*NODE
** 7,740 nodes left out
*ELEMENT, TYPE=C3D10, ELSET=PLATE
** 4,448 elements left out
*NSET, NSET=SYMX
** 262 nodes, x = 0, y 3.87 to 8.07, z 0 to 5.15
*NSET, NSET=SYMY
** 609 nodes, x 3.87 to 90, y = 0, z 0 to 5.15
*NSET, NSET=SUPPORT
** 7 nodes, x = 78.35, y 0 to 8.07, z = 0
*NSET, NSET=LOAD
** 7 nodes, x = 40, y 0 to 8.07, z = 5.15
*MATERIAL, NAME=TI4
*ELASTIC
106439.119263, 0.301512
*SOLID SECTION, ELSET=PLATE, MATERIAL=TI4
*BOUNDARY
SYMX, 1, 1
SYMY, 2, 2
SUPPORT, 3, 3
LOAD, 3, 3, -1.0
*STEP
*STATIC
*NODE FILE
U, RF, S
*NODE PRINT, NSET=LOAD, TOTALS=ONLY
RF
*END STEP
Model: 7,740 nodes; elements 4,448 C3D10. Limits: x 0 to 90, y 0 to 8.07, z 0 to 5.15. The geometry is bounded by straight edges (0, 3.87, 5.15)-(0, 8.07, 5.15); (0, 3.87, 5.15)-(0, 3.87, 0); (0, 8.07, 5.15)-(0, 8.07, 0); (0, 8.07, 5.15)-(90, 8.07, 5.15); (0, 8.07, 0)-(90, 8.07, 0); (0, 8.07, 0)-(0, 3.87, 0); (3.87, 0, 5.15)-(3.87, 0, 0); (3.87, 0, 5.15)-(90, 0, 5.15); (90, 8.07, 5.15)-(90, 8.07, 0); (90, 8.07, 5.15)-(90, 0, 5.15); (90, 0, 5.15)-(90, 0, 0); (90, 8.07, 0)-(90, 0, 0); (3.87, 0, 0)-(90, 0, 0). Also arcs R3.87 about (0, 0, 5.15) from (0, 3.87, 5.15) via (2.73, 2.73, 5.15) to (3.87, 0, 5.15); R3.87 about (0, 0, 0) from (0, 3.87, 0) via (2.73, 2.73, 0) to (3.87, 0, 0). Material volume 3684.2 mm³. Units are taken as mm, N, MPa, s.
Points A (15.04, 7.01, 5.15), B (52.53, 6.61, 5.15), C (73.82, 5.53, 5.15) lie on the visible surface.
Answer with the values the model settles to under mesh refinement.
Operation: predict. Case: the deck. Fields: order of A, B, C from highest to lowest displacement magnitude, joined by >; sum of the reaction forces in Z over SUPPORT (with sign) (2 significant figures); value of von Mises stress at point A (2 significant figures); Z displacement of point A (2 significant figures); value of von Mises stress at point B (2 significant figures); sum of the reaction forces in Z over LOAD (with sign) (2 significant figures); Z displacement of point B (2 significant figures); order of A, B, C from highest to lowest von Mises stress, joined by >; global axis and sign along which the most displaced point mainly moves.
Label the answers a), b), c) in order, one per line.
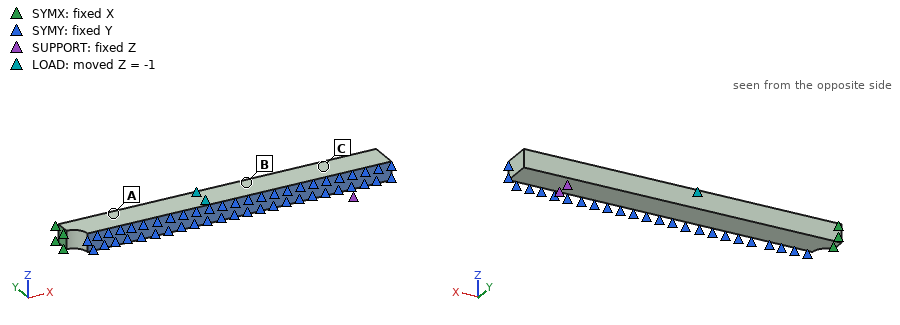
a) A > B > C
b) 120 N
c) 130 MPa
d) -1.4 mm
e) 85 MPa
f) -120 N
g) -0.72 mm
h) A > B > C
i) -Z
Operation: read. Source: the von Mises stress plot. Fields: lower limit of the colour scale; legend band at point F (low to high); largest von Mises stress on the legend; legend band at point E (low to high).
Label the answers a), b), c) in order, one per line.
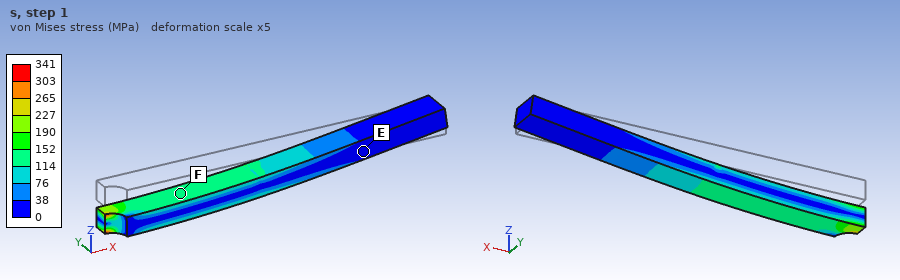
a) 0 MPa
b) 114 to 152 MPa
c) 341 MPa
d) 0 to 38 MPa
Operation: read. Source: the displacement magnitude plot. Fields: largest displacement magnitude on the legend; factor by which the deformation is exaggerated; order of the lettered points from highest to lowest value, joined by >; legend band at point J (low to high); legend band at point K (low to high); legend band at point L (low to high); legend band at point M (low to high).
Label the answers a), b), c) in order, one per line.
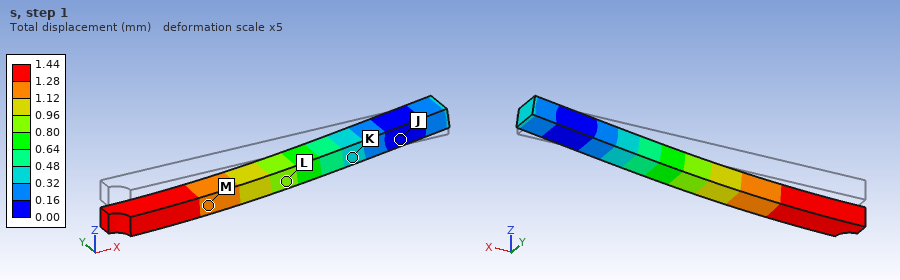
a) 1.44 mm
b) 5
c) M > L > K > J
d) 0.00 to 0.16 mm
e) 0.32 to 0.48 mm
f) 0.80 to 0.96 mm
g) 1.12 to 1.28 mm
